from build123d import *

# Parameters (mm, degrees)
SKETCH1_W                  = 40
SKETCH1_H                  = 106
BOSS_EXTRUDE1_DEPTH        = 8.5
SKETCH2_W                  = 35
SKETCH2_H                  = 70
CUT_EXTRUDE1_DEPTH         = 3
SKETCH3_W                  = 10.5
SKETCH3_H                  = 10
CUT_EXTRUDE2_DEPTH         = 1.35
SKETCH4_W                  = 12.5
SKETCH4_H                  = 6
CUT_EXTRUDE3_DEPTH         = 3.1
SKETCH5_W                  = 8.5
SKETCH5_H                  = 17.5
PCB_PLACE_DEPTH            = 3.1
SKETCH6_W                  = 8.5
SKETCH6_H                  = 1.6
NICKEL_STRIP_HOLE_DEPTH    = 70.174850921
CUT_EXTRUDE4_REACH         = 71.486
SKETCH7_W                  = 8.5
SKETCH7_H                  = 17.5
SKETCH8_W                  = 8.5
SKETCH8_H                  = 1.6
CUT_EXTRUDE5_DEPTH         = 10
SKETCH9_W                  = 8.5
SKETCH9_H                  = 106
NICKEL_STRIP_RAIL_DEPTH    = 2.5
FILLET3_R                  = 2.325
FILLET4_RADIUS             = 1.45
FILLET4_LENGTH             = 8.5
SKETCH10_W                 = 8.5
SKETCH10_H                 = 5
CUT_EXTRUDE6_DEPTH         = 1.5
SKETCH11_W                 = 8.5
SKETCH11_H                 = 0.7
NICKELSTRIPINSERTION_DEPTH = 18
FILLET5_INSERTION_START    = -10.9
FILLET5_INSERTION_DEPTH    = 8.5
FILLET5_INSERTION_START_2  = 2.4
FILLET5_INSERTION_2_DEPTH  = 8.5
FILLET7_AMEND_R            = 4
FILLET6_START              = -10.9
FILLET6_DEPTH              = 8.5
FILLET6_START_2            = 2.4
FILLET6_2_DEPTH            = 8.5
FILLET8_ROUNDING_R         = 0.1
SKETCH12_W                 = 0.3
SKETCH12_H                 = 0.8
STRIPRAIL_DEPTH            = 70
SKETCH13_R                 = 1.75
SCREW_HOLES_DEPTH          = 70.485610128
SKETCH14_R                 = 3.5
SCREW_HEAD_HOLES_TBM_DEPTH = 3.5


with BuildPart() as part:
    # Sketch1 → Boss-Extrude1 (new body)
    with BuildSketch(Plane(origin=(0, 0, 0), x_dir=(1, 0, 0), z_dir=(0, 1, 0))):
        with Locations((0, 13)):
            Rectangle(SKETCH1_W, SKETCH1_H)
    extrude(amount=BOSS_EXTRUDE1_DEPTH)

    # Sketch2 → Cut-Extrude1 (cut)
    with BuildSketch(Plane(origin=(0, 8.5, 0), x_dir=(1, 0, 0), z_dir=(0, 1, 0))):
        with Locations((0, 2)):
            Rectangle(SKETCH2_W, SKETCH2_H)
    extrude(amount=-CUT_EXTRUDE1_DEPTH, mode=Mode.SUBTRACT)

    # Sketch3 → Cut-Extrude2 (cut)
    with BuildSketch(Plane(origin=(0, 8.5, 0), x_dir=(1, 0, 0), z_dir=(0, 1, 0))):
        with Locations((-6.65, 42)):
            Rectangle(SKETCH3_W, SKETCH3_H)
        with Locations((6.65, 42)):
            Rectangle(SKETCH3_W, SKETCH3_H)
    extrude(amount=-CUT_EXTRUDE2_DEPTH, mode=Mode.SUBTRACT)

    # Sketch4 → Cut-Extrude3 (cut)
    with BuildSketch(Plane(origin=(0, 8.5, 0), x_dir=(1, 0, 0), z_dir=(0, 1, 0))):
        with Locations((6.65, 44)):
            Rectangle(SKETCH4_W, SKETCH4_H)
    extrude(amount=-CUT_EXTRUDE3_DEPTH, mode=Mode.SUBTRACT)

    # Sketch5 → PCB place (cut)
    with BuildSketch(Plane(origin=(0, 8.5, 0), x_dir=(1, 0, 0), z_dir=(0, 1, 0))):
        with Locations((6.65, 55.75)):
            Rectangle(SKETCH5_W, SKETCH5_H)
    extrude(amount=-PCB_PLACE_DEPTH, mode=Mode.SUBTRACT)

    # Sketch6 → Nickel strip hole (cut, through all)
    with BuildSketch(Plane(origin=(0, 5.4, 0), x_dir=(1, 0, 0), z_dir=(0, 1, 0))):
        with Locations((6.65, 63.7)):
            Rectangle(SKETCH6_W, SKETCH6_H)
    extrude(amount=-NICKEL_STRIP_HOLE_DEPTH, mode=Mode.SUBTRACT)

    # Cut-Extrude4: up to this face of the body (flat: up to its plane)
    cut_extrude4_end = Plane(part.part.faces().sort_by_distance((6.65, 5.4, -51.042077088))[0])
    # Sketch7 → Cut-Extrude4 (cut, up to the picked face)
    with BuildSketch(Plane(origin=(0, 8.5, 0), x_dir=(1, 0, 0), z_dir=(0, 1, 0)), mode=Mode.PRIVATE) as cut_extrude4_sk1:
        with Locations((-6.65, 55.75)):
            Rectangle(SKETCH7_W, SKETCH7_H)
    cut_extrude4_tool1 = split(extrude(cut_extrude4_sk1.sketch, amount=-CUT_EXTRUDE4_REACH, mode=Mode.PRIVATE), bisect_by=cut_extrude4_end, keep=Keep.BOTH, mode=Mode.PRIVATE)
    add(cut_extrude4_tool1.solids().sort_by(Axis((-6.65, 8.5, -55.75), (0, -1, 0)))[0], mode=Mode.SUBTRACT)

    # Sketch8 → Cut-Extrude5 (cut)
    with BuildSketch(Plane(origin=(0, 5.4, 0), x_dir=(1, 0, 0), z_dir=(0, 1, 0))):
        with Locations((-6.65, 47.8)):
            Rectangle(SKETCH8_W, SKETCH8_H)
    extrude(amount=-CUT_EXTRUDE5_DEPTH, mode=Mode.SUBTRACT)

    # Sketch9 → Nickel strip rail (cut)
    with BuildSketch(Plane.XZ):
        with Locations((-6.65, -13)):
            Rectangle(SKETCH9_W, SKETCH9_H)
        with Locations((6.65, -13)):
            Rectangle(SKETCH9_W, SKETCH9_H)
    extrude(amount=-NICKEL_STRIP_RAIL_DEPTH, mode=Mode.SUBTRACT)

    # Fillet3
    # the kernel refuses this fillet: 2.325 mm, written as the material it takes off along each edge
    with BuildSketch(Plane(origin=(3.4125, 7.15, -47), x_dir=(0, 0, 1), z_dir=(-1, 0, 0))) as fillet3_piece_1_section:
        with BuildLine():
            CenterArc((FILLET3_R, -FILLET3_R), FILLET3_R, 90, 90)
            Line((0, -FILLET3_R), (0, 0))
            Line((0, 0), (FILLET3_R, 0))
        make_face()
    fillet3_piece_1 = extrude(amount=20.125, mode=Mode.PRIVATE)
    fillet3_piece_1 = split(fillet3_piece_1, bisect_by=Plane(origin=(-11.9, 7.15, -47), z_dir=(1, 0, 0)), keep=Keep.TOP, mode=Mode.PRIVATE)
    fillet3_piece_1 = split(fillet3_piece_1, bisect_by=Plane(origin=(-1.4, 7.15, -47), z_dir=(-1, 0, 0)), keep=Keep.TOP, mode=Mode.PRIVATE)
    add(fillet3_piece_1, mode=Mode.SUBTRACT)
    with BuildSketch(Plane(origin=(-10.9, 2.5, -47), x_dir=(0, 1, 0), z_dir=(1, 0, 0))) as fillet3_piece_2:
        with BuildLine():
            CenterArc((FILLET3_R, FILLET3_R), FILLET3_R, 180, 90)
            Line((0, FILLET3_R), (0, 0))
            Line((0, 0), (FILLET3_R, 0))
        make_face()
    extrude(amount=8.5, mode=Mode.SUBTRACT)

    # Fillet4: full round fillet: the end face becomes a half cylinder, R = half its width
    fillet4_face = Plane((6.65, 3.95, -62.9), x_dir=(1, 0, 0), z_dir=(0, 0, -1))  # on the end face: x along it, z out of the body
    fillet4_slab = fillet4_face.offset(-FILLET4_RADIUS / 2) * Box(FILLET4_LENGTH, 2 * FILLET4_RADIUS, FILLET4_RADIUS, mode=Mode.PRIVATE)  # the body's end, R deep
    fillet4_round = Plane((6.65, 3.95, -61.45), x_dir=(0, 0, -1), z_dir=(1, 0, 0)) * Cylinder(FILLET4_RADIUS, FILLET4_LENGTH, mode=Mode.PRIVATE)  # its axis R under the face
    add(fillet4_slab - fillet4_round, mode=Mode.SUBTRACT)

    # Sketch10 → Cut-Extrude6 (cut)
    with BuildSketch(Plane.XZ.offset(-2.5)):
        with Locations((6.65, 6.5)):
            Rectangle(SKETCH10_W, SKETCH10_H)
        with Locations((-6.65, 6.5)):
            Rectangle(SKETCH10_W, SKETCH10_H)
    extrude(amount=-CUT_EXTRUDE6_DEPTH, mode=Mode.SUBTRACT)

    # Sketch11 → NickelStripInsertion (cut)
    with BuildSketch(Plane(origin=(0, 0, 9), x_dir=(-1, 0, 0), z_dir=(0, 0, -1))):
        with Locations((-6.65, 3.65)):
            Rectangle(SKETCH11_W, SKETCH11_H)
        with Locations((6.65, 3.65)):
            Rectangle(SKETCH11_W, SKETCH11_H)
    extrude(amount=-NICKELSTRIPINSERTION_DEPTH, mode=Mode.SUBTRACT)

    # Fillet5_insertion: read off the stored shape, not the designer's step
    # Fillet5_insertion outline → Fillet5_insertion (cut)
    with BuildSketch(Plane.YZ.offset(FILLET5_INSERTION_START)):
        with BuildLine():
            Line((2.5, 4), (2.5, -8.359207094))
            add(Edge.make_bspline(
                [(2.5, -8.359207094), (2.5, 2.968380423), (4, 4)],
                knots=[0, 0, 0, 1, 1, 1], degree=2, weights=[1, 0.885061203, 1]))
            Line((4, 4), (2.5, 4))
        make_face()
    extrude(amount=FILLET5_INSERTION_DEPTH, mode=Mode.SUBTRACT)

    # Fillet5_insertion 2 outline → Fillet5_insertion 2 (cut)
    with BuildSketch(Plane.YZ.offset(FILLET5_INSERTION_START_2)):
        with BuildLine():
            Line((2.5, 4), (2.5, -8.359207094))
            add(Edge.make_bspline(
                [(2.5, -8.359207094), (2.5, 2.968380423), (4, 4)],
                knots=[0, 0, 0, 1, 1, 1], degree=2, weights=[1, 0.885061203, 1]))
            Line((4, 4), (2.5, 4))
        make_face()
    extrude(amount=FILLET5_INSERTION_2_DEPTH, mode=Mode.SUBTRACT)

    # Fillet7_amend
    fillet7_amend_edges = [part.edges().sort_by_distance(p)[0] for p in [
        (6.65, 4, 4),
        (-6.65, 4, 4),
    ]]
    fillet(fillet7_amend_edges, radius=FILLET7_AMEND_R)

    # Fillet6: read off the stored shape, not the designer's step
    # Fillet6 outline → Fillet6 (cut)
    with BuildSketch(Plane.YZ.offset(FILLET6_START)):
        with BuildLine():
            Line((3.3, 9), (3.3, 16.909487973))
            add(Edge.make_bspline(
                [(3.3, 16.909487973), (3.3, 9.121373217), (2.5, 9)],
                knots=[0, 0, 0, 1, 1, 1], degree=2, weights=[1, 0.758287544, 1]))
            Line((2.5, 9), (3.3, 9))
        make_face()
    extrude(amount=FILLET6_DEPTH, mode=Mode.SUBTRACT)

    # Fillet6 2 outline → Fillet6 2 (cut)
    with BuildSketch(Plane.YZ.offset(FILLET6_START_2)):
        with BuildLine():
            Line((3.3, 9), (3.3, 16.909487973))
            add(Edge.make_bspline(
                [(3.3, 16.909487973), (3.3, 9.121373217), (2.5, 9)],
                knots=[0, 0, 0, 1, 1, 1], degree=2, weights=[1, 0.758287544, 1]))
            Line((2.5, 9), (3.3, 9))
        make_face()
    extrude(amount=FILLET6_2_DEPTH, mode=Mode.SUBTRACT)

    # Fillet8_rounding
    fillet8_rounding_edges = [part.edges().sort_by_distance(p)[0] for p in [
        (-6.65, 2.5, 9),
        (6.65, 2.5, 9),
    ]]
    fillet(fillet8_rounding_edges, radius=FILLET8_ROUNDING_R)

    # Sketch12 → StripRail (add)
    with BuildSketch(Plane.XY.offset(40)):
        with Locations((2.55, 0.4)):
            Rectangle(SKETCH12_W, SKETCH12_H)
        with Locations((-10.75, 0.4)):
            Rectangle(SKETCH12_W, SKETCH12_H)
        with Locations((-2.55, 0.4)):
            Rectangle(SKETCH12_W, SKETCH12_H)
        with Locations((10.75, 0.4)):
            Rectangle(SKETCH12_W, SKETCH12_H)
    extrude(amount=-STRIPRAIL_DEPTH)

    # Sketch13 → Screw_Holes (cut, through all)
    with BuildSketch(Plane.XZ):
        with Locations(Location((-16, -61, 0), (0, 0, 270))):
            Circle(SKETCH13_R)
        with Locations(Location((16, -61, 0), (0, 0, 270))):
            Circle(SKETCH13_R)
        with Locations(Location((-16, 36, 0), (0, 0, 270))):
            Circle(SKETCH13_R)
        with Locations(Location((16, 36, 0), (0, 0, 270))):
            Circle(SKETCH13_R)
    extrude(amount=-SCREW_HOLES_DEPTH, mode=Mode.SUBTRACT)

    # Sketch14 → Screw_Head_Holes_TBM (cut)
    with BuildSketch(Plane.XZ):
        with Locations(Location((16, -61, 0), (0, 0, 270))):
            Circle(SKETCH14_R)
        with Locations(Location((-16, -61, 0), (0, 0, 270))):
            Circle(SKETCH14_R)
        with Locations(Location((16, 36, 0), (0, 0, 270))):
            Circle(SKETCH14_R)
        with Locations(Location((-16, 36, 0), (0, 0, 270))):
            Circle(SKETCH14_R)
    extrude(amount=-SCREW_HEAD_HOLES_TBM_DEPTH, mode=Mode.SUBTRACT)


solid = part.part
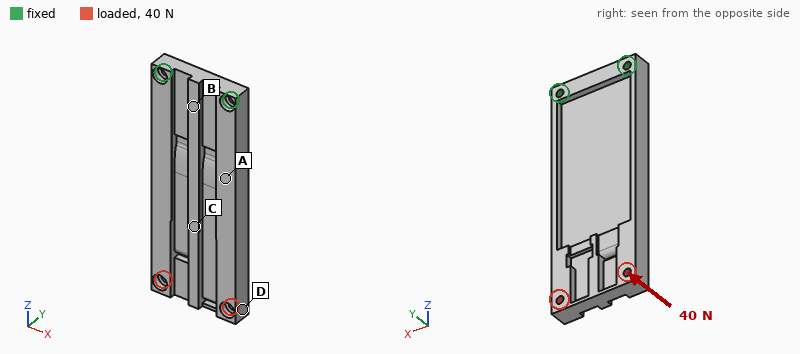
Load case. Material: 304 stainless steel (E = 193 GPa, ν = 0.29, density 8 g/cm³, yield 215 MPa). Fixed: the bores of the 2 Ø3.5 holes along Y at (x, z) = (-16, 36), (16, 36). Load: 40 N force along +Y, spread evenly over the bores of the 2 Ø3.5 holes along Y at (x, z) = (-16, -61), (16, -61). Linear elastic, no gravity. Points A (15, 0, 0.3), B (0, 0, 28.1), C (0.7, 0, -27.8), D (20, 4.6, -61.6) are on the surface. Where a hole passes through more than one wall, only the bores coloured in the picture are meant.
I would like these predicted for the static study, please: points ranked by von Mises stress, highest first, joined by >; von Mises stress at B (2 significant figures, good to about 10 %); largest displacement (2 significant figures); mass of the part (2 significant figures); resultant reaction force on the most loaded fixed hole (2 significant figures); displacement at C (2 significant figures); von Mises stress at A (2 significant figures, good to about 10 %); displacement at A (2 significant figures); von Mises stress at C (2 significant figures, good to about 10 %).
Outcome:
B > A > C > D
17 MPa
0.13 mm
170 g
21 N
0.068 mm
13 MPa
0.028 mm
7.1 MPa
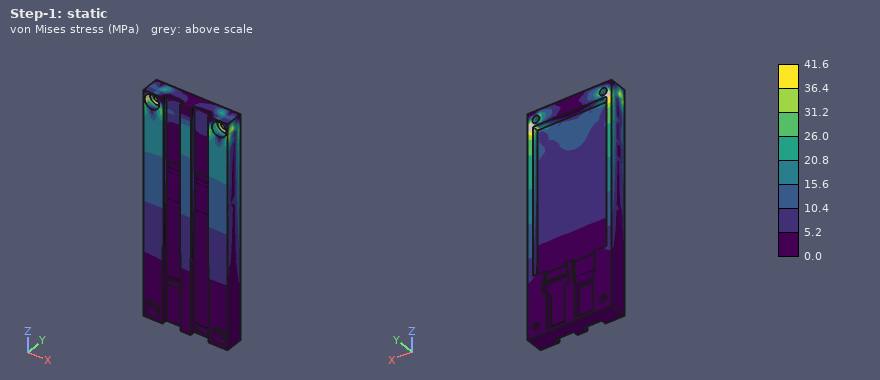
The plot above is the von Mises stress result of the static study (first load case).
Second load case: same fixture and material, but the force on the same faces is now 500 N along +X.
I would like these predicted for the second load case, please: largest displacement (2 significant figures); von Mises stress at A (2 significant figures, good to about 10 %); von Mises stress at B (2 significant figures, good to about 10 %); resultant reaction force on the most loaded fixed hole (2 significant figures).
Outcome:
53 µm
15 MPa
8.2 MPa
1.5 kN
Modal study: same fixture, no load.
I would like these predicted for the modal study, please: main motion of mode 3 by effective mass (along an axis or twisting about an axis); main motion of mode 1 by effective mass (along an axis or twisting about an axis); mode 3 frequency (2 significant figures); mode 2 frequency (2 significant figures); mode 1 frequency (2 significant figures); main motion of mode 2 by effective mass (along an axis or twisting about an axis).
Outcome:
along X
along Y
2400 Hz
1500 Hz
390 Hz
twisting about Z
